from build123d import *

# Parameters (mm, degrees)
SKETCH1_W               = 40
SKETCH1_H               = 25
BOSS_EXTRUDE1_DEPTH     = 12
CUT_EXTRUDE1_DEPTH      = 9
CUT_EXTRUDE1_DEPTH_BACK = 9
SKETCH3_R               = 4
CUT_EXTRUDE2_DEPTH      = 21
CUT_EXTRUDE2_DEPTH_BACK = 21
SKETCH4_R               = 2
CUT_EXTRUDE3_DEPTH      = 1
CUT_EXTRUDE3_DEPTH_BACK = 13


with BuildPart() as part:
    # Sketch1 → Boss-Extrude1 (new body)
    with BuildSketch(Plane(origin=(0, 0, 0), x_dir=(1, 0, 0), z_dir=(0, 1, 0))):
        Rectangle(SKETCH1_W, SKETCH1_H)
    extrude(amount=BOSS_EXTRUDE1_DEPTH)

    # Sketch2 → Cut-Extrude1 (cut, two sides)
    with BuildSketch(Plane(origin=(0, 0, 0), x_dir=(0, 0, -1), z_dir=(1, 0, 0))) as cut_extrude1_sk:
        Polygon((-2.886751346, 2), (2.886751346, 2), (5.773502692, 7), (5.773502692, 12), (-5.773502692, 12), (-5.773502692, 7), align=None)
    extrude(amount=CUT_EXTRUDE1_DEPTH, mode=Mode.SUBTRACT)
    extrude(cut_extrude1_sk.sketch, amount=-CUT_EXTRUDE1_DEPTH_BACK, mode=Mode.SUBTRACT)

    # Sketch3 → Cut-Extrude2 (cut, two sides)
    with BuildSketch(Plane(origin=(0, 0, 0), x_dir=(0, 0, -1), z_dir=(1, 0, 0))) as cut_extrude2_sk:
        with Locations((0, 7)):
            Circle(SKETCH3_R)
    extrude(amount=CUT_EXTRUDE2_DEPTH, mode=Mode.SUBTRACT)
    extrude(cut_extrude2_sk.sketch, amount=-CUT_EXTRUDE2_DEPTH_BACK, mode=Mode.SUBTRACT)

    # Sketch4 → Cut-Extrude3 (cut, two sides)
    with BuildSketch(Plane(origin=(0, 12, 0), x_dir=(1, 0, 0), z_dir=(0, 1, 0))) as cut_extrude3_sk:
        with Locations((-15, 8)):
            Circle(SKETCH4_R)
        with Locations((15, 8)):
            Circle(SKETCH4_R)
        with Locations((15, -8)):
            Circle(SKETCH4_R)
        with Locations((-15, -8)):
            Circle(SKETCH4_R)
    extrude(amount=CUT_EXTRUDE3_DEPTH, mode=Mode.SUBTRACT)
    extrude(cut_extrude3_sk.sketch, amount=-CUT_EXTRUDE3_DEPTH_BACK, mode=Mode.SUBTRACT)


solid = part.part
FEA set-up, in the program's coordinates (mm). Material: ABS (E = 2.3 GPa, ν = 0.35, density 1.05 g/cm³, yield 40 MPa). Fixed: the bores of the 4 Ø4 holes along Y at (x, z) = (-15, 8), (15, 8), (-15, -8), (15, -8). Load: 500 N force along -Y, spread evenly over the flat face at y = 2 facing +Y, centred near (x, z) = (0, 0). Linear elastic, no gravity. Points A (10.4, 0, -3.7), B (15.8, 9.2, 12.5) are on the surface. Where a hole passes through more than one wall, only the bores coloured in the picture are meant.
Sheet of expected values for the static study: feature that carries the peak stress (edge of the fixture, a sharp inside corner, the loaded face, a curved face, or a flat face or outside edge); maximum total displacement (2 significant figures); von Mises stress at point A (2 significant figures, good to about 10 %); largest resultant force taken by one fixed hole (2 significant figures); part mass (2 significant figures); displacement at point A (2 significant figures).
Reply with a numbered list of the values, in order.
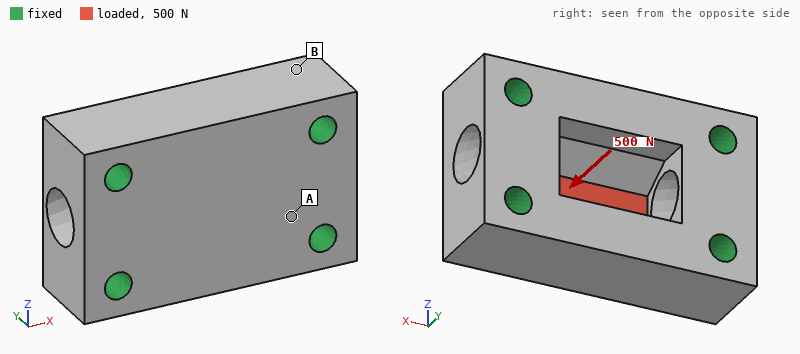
1. a flat face or outside edge
2. 0.10 mm
3. 4.6 MPa
4. 140 N
5. 8.9 g
6. 0.018 mm
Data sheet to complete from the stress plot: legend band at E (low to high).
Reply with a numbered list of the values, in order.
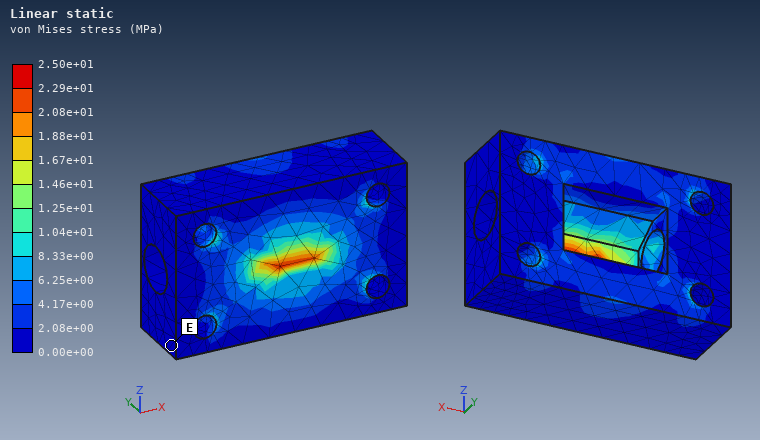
1. 0.00e+00 to 2.08e+00 MPa
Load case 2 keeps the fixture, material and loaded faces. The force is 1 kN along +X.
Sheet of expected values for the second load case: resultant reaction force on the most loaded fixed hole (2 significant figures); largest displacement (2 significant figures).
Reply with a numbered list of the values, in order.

1. 270 N
2. 69 µm
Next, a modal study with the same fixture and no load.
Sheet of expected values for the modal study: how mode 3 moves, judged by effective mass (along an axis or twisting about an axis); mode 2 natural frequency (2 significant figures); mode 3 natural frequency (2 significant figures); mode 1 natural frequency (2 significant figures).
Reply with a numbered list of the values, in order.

1. along Y
2. 12 kHz
3. 13 kHz
4. 12 kHz
